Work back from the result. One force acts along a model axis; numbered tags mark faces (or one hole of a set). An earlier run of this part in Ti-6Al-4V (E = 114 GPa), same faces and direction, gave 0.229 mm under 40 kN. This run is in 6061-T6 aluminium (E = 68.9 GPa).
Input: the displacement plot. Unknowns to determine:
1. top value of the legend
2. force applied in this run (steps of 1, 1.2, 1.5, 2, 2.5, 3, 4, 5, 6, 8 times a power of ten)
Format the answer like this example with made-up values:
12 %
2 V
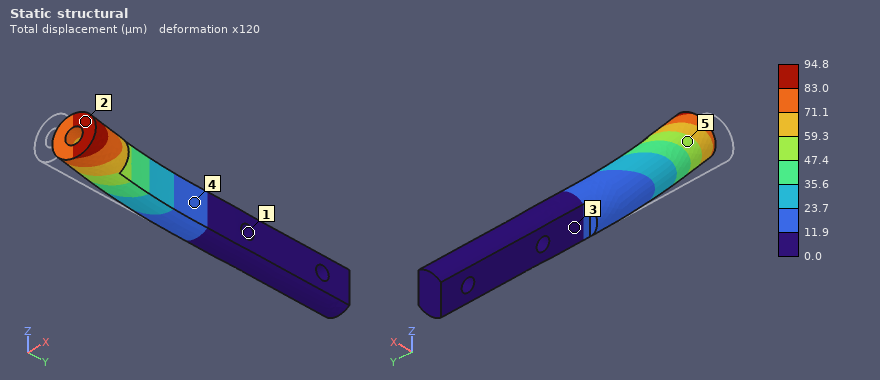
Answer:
94.8 µm
10 kN
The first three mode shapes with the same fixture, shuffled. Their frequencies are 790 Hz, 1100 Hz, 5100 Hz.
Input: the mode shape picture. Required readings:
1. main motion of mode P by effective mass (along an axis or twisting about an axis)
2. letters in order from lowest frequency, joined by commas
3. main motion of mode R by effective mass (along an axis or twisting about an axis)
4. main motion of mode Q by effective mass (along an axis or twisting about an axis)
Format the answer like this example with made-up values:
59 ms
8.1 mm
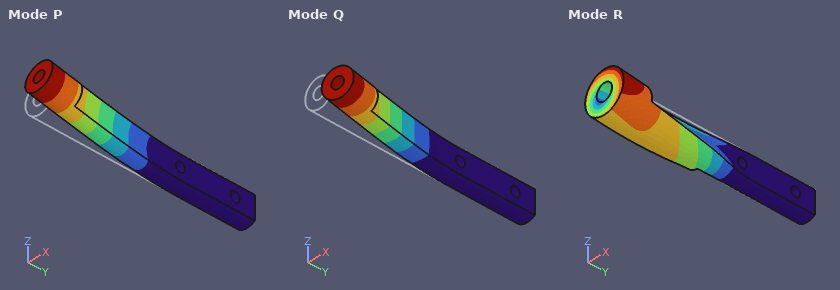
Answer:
along Z
Q, P, R
twisting about Y
along X
